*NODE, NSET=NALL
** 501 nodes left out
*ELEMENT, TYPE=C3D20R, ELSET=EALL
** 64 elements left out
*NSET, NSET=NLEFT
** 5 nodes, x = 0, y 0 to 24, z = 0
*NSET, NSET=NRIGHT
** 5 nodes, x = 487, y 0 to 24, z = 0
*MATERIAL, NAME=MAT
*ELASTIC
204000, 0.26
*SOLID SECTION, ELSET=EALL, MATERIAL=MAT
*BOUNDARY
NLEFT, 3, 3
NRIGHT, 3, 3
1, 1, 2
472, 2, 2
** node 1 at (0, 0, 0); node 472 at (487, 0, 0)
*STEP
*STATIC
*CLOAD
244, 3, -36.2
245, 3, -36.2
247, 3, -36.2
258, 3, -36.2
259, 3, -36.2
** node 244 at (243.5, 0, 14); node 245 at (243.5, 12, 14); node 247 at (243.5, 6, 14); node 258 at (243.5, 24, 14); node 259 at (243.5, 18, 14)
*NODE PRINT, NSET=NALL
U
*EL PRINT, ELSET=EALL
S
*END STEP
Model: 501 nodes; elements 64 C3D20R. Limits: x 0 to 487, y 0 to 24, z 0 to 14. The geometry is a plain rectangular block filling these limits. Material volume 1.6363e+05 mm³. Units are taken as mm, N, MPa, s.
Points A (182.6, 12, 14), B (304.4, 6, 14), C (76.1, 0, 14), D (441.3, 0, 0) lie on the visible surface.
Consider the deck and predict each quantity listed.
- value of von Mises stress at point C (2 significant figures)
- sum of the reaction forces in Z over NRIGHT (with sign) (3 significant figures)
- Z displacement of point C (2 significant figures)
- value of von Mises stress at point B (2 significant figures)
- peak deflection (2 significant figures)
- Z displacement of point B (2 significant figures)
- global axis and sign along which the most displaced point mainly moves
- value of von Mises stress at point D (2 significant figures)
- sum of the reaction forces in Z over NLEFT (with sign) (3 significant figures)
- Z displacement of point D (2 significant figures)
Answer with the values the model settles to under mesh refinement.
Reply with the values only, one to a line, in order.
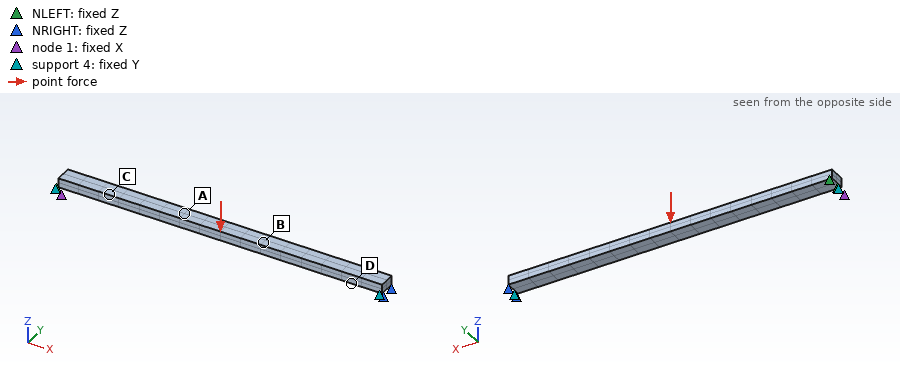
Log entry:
8.8 MPa
90.5 N
-0.18 mm
21 MPa
0.39 mm
-0.36 mm
-Z
5.3 MPa
90.5 N
-0.11 mm
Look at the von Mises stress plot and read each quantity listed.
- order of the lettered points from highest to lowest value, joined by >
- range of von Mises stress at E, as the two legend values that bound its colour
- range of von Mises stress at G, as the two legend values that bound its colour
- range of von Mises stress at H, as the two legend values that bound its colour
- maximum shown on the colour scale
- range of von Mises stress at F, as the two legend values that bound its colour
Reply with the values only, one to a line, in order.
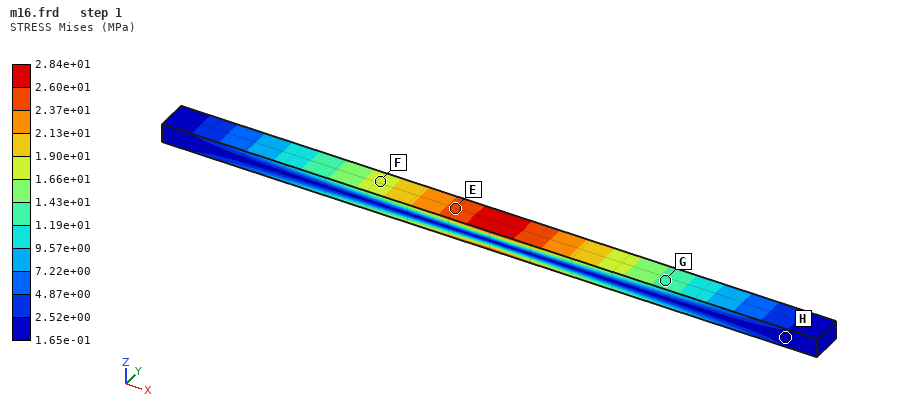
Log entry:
E > F > G > H
2.37e+01 to 2.60e+01 MPa
1.19e+01 to 1.43e+01 MPa
1.65e-01 to 2.52e+00 MPa
2.84e+01 MPa
1.66e+01 to 1.90e+01 MPa
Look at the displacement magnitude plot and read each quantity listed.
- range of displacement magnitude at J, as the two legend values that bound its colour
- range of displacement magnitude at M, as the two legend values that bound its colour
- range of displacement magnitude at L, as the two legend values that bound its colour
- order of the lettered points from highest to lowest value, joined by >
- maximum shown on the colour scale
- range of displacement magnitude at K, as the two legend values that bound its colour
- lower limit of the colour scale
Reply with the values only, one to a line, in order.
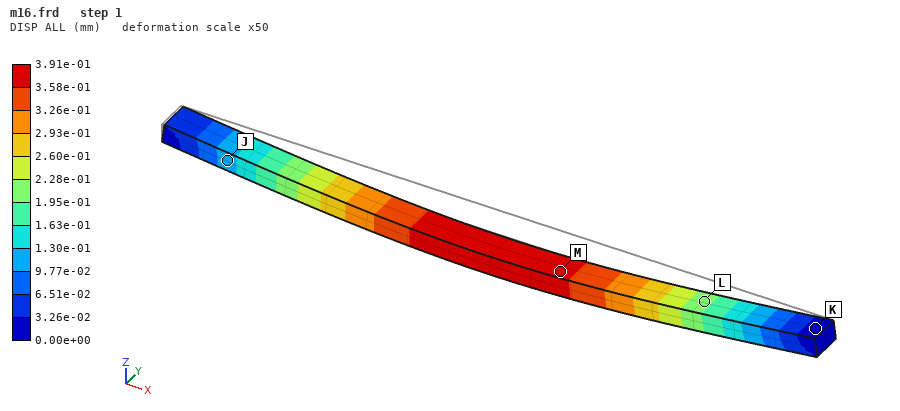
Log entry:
9.77e-02 to 1.30e-01 mm
3.58e-01 to 3.91e-01 mm
1.95e-01 to 2.28e-01 mm
M > L > J > K
3.91e-01 mm
0.00e+00 to 3.26e-02 mm
0.00e+00 mm
